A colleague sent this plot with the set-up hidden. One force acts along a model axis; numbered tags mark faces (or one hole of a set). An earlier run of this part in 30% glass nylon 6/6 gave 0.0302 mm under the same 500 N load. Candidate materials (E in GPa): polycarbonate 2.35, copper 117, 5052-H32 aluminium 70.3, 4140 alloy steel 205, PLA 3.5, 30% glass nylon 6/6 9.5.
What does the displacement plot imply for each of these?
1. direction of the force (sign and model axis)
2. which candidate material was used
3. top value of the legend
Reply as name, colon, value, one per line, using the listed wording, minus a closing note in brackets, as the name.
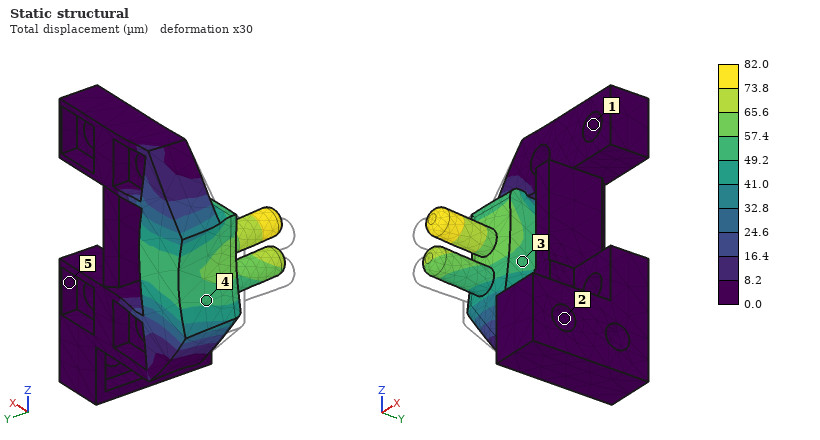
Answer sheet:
direction of the force: +X
which candidate material was used: PLA
top value of the legend: 82.0 µm
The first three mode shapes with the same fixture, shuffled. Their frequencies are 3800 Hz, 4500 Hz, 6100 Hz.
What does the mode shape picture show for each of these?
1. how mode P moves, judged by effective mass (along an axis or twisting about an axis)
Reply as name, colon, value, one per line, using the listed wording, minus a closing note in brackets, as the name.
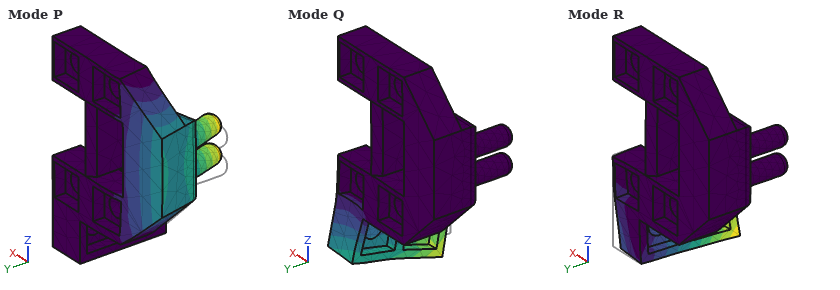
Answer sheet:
how mode P moves, judged by effective mass: along Y
